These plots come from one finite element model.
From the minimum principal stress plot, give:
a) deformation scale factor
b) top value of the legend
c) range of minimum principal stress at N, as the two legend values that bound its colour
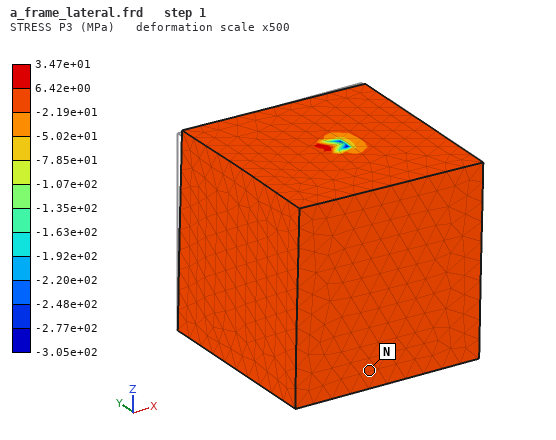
500
3.47e+01 MPa
-2.19e+01 to 6.42e+00 MPa
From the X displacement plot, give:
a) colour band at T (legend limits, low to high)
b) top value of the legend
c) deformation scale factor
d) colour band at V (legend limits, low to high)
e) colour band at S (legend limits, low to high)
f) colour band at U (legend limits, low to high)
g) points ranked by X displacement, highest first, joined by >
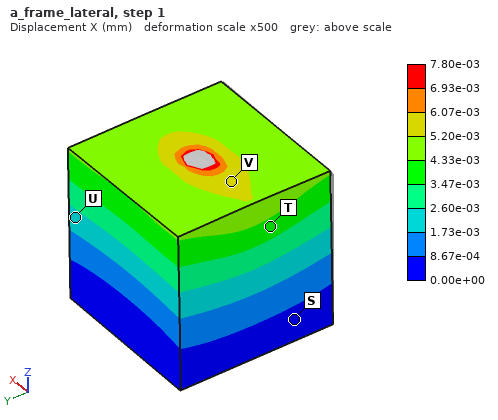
3.47e-03 to 4.33e-03 mm
7.80e-03 mm
500
5.20e-03 to 6.07e-03 mm
0.00e+00 to 8.67e-04 mm
1.73e-03 to 2.60e-03 mm
V > T > U > S
